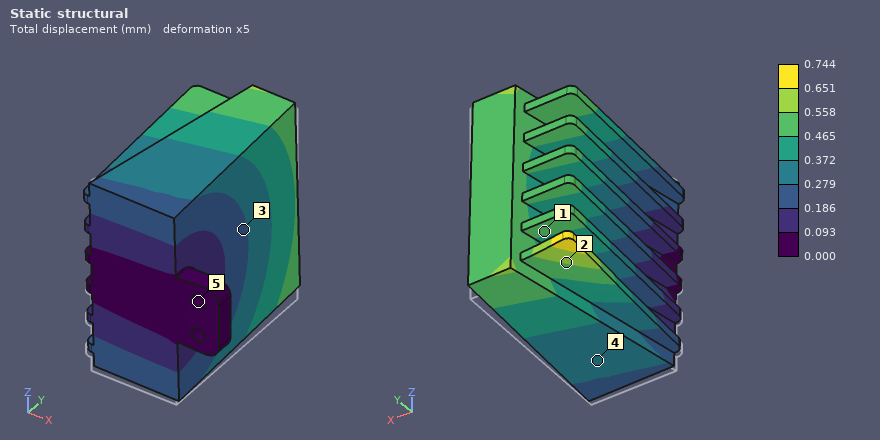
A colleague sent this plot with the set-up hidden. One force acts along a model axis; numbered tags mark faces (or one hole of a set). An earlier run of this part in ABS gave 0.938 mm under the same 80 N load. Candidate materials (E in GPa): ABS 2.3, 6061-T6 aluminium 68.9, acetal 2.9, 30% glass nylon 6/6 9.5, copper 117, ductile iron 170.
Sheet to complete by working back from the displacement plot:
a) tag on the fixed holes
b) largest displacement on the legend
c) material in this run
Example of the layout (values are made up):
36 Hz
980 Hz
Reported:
5
0.744 mm
acetal
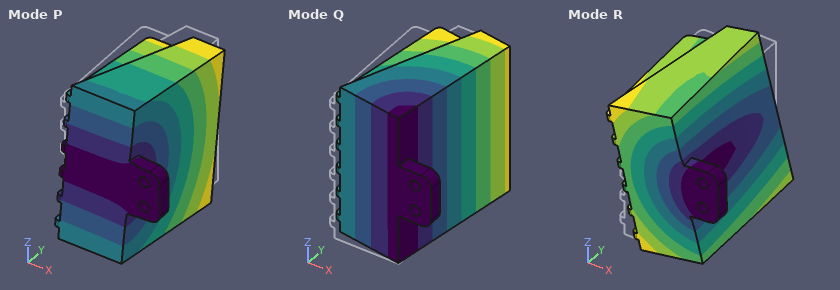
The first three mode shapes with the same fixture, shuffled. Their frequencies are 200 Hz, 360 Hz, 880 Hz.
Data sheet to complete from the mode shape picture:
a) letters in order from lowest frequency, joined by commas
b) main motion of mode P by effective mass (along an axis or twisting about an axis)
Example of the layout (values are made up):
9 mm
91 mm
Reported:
Q, P, R
along Z
